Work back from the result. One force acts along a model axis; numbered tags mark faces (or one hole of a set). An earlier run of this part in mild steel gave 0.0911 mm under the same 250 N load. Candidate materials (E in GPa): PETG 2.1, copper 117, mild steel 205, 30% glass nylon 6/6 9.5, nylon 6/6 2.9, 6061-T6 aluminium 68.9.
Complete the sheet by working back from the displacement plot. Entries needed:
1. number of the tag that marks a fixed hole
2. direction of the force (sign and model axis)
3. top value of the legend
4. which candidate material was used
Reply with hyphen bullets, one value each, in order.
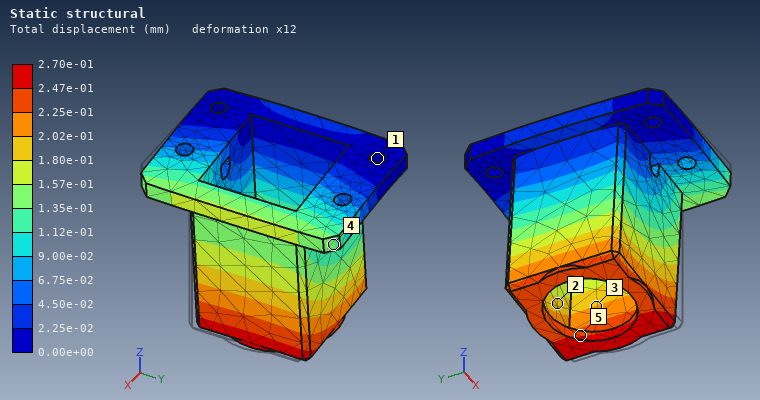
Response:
- 1
- -X
- 2.70e-01 mm
- 6061-T6 aluminium
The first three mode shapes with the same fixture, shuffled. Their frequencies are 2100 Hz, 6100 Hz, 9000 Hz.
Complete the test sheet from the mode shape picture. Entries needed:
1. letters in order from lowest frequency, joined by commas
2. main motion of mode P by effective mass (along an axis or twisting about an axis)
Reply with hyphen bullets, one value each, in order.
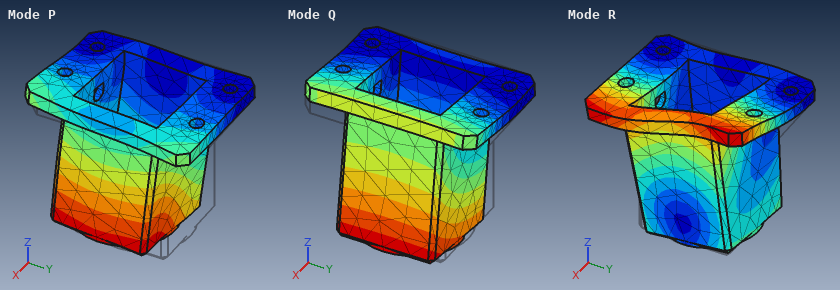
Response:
- Q, P, R
- along Y
